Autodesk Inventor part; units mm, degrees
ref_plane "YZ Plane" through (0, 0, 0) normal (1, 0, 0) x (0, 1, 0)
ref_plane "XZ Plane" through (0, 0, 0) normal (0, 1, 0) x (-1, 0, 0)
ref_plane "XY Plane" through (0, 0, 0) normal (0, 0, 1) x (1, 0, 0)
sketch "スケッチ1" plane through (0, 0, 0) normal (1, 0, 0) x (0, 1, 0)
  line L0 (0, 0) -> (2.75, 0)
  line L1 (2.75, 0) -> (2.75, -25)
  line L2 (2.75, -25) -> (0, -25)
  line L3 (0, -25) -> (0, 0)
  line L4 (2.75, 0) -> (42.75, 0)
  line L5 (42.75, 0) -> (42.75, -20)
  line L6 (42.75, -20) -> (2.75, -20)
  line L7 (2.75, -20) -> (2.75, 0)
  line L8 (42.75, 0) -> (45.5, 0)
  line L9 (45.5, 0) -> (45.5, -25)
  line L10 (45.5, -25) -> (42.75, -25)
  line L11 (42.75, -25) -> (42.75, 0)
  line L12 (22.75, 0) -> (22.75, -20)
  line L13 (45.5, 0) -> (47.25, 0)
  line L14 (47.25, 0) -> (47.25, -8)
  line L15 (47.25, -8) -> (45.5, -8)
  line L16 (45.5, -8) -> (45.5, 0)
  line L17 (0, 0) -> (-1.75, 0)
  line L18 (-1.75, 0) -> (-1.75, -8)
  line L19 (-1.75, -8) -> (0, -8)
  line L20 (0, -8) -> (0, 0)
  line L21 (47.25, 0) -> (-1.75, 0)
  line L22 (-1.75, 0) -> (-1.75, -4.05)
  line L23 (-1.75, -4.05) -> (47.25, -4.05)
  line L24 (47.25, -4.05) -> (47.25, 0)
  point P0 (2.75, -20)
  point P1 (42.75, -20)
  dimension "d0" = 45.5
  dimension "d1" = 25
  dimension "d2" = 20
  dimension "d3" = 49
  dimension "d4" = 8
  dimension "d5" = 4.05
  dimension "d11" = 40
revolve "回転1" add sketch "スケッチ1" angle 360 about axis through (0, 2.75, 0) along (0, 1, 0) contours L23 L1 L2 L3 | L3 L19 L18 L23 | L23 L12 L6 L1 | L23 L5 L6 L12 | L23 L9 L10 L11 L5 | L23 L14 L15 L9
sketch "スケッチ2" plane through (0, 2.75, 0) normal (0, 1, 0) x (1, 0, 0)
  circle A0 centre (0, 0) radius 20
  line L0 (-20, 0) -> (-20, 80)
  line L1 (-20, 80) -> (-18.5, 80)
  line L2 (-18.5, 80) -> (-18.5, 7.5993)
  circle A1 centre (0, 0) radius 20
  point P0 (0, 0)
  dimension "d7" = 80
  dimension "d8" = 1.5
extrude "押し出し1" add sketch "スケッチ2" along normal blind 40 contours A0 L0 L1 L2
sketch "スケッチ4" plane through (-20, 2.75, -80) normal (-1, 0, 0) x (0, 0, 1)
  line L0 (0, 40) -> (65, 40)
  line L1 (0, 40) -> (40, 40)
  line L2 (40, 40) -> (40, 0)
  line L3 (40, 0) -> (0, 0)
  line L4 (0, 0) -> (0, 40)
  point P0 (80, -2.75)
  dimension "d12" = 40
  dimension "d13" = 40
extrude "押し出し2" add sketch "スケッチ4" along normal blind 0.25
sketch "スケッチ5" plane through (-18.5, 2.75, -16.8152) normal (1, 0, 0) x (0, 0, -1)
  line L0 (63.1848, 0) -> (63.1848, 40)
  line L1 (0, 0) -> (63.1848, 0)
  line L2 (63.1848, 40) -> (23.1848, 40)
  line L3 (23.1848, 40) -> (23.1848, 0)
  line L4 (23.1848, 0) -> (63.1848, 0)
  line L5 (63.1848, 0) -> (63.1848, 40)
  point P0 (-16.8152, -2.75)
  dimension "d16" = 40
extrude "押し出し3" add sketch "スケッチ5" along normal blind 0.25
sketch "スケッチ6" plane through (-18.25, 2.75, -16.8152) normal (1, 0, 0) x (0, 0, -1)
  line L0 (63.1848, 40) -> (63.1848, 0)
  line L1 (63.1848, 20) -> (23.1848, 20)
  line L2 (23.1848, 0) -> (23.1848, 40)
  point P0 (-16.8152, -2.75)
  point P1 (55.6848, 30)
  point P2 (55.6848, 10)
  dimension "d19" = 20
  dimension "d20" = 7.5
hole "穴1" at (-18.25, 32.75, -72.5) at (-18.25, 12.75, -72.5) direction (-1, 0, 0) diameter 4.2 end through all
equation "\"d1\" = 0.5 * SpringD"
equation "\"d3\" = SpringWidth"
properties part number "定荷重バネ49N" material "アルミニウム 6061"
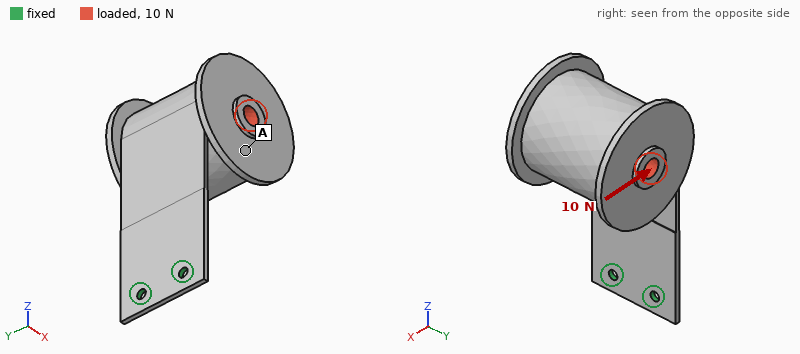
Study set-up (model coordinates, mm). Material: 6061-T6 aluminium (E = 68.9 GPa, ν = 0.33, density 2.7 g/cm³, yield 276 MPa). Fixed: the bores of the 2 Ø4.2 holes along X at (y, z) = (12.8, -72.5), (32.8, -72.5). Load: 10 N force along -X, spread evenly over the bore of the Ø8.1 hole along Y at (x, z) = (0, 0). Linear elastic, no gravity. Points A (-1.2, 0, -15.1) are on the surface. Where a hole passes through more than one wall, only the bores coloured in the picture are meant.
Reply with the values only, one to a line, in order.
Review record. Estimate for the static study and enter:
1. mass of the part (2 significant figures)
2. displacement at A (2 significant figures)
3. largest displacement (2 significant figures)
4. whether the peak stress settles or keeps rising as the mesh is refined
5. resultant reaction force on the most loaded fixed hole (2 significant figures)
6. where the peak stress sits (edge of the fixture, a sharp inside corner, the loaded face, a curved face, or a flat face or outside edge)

170 g
0.61 mm
1.3 mm
keeps rising
5.0 N
edge of the fixture
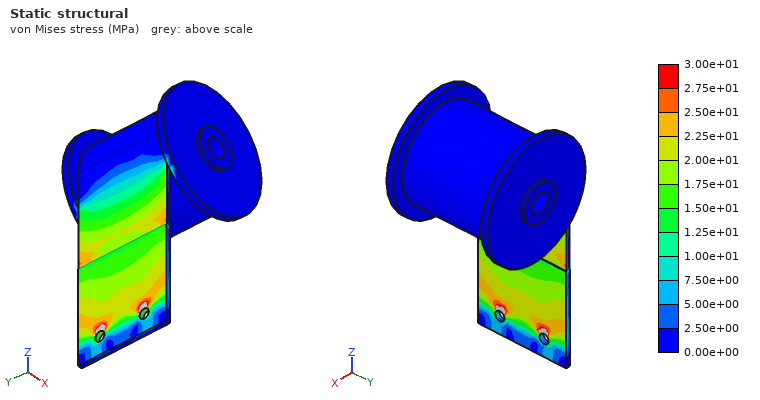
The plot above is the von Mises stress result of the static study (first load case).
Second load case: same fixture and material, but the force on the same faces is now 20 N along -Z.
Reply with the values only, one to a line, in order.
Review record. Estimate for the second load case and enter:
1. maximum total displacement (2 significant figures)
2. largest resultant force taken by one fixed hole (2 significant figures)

1.3 mm
10 N
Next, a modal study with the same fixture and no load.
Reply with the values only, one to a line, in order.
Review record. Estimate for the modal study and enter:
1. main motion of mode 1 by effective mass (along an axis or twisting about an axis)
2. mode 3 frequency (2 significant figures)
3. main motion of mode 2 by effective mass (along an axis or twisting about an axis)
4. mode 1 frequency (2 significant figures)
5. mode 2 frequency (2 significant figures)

along X
190 Hz
along Y
38 Hz
100 Hz
